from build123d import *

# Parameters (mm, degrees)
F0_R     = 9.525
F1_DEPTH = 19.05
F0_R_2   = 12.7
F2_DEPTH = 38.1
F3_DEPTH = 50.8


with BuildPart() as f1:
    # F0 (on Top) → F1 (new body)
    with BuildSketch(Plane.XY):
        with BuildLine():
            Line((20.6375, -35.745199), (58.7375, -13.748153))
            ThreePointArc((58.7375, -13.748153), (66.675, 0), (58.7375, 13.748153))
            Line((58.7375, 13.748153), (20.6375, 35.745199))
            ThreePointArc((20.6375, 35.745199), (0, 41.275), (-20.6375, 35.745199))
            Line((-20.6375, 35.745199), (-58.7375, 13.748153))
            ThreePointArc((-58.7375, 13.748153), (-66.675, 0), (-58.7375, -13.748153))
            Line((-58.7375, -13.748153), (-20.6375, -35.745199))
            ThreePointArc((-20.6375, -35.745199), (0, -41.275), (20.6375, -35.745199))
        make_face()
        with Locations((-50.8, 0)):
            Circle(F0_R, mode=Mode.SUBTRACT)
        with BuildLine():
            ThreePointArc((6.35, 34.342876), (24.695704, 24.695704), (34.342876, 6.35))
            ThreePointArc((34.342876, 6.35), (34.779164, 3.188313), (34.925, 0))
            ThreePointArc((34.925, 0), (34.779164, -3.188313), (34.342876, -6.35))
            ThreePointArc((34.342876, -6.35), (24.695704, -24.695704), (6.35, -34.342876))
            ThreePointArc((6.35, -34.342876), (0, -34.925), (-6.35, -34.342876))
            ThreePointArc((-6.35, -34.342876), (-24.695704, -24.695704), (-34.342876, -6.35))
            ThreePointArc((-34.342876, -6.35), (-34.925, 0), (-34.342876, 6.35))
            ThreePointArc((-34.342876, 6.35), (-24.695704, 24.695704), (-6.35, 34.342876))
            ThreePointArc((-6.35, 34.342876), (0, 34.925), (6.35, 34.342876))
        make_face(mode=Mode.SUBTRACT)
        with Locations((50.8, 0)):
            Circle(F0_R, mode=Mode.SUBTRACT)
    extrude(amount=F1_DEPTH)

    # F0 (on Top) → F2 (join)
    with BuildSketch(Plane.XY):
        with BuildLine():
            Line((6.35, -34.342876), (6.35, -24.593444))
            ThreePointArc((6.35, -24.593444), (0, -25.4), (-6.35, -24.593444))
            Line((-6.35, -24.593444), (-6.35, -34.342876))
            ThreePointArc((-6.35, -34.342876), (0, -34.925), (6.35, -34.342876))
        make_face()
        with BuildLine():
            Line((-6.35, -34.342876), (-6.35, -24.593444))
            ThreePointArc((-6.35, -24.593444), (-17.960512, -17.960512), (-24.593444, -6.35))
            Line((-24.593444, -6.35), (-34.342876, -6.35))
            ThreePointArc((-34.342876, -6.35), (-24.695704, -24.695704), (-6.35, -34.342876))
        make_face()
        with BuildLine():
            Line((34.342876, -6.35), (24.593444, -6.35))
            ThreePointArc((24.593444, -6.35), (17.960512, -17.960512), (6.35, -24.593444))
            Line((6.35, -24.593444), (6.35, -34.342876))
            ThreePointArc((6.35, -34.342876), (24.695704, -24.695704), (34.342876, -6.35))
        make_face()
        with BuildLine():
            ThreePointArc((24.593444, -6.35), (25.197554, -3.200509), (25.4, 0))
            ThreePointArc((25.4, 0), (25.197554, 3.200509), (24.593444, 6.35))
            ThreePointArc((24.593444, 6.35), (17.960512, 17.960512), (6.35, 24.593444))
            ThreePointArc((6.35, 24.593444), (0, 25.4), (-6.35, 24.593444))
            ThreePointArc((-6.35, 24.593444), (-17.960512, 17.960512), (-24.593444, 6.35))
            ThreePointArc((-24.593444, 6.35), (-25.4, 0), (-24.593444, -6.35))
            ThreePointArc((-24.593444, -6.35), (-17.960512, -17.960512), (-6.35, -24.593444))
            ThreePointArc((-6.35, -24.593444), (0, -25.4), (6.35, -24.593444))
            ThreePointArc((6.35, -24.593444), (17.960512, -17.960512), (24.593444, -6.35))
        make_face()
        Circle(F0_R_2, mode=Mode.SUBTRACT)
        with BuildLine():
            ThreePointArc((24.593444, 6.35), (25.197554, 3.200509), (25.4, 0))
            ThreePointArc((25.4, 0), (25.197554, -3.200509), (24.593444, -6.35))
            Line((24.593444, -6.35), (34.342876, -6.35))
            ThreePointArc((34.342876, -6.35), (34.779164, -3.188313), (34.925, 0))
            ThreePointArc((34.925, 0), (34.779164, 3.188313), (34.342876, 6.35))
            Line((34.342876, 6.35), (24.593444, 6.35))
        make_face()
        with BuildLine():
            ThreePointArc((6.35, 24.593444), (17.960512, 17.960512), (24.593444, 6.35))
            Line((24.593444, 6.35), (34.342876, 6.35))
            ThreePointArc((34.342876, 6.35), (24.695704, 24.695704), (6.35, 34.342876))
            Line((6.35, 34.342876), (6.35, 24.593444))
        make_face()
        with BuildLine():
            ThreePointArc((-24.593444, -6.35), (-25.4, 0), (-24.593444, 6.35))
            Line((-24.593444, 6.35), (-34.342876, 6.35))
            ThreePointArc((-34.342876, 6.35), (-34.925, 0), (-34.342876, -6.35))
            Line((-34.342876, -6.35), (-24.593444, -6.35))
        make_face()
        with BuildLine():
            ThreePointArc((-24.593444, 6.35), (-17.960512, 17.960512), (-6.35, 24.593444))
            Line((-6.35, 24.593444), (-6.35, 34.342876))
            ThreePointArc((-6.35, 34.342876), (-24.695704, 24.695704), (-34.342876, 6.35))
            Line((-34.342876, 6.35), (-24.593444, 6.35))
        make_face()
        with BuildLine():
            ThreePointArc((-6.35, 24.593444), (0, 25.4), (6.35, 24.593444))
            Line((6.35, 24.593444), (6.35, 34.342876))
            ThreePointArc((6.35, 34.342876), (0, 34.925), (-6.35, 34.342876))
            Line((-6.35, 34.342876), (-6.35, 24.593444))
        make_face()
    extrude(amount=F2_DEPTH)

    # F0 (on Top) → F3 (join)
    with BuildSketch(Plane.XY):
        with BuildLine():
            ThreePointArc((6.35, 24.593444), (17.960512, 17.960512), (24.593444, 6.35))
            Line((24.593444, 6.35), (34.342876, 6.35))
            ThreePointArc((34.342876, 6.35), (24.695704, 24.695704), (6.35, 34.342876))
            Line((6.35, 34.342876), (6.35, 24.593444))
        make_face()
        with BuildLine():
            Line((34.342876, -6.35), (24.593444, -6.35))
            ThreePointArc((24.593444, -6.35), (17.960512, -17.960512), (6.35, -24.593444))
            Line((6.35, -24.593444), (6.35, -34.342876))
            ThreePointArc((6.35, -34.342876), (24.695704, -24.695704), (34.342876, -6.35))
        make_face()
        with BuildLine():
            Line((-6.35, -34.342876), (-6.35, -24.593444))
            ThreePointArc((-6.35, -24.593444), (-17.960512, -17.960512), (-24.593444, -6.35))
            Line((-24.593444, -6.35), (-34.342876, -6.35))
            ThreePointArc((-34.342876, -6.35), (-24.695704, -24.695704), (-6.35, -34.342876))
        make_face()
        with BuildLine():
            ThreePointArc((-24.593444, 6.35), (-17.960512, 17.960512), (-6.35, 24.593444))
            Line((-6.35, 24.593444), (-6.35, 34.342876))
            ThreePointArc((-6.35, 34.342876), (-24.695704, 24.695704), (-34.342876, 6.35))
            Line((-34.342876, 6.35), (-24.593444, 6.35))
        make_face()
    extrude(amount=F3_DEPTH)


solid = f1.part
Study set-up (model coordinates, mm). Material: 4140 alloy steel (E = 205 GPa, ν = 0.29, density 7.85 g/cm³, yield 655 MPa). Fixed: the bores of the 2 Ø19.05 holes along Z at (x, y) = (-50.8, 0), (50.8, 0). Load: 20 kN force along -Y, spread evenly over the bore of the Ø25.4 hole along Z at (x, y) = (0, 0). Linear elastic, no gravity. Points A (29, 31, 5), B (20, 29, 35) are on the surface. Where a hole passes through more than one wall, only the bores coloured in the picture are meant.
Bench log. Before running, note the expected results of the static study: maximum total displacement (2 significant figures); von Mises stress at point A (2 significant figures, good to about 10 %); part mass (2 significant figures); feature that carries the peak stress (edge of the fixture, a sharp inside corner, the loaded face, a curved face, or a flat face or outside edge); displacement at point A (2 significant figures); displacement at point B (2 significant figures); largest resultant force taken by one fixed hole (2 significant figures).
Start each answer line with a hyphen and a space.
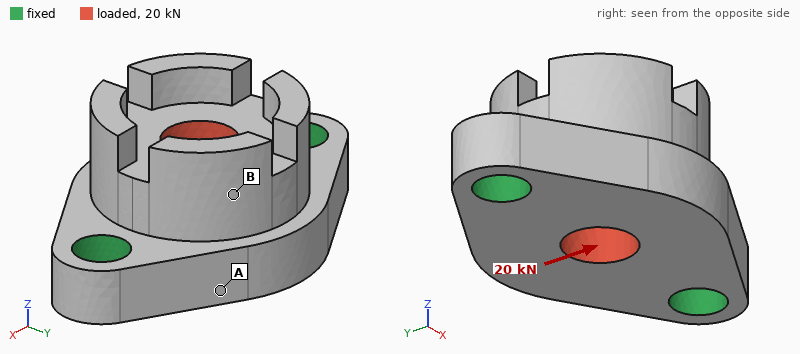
- 16 µm
- 17 MPa
- 1.6 kg
- edge of the fixture
- 6.3 µm
- 12 µm
- 10 kN
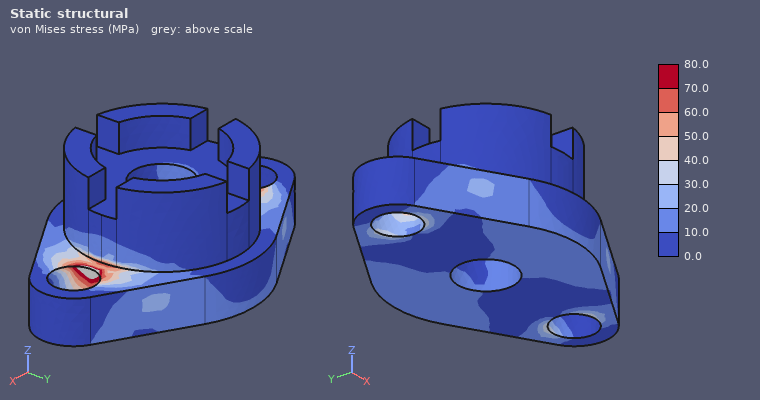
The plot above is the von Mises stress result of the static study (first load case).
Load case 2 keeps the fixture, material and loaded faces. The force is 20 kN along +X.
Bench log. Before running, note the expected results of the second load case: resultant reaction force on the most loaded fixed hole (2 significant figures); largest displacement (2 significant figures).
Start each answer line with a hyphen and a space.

- 10 kN
- 3.1 µm
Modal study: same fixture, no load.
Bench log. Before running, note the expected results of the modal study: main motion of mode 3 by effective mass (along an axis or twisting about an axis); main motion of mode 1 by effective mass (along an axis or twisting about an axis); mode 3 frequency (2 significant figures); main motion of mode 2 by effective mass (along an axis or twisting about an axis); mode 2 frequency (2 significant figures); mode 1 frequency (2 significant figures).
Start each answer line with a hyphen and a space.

- along Y
- along Y
- 11 kHz
- along Z
- 7500 Hz
- 4600 Hz
